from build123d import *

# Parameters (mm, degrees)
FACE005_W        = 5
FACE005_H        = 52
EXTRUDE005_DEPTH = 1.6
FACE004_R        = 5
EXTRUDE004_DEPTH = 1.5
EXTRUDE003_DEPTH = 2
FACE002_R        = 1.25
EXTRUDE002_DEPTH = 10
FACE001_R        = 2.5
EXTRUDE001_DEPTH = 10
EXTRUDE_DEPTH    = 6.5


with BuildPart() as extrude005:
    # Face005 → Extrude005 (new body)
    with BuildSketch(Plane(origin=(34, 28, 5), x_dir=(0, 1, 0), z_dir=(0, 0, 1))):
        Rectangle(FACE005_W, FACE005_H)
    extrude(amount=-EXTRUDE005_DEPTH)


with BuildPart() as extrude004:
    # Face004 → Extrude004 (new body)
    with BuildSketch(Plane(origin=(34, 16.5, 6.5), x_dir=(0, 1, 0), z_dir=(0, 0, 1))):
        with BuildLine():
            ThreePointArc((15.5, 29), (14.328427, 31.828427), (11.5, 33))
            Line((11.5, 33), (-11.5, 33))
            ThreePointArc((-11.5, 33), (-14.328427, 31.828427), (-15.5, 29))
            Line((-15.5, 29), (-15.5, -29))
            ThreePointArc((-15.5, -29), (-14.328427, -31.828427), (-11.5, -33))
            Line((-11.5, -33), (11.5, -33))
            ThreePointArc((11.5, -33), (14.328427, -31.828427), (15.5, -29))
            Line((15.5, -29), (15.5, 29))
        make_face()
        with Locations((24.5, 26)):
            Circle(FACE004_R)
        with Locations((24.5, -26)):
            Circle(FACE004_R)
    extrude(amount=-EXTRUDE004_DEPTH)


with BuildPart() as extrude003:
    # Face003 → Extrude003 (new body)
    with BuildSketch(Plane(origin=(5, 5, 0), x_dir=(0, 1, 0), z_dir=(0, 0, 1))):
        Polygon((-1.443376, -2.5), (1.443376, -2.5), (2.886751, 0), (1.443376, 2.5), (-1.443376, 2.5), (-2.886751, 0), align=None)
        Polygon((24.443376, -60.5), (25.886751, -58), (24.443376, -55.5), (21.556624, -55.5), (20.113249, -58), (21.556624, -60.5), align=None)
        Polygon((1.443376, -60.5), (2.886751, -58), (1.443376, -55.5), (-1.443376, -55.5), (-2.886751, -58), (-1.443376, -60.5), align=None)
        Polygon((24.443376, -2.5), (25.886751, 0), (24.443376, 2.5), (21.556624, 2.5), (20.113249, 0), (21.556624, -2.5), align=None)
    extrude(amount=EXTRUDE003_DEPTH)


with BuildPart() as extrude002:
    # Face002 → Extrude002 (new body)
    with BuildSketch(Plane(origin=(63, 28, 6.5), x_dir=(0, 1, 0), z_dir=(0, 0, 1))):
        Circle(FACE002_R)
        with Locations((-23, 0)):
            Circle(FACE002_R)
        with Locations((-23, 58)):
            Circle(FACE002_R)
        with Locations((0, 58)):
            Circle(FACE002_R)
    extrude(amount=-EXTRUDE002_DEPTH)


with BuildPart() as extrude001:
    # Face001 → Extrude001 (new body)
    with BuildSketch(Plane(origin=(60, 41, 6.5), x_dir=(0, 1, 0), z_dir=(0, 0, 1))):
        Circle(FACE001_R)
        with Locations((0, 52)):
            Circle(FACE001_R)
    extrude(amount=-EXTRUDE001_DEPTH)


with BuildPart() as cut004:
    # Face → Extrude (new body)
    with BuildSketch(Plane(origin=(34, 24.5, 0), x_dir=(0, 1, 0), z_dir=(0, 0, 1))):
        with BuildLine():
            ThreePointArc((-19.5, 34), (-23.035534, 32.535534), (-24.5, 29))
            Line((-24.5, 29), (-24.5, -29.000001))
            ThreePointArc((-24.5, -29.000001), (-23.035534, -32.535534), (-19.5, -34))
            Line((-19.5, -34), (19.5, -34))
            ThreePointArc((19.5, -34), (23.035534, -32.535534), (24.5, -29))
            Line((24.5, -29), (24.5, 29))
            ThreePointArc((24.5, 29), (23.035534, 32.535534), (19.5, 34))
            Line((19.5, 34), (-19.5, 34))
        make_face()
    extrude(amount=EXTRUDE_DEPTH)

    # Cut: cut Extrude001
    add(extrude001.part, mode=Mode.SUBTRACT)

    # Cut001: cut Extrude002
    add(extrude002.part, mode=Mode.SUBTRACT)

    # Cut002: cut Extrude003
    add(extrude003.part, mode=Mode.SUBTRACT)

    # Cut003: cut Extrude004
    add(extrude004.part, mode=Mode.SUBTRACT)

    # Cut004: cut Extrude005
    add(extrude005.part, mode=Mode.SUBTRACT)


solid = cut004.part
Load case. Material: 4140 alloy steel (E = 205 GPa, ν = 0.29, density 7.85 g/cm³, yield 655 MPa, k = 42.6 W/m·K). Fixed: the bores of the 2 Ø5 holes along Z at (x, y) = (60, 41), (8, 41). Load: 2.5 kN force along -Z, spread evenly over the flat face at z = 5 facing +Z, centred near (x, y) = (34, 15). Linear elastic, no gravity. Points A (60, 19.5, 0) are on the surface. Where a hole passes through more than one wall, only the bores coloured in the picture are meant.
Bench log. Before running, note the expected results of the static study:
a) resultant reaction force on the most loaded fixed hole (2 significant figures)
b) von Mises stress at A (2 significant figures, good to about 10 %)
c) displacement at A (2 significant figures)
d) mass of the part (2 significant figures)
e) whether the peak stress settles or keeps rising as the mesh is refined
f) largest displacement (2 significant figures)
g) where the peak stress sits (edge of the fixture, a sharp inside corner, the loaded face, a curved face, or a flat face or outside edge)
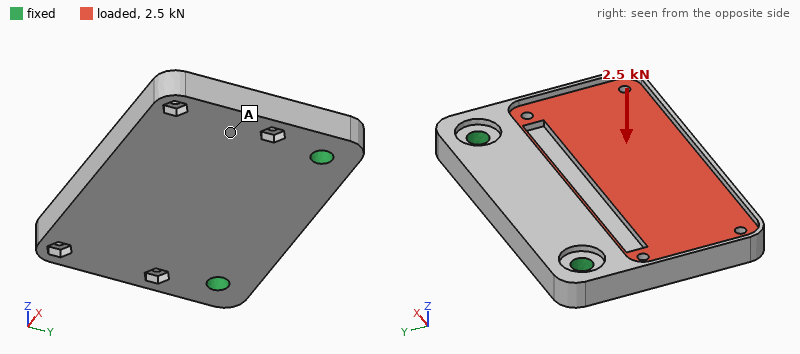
1.3 kN
59 MPa
0.100 mm
140 g
keeps rising
0.29 mm
edge of the fixture
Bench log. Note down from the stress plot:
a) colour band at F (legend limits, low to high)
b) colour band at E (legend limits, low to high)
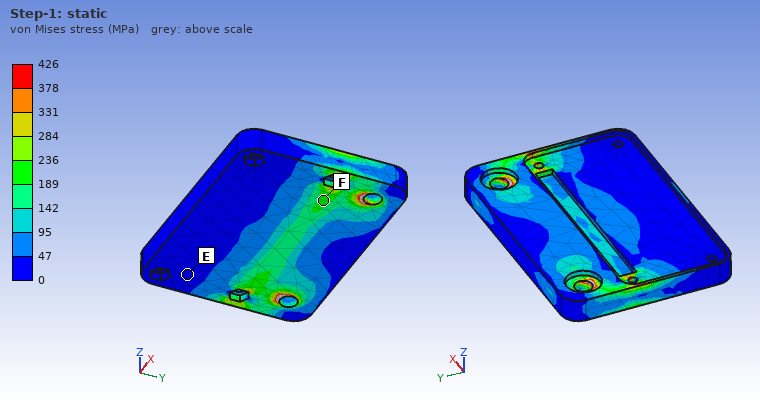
189 to 236 MPa
0 to 47 MPa
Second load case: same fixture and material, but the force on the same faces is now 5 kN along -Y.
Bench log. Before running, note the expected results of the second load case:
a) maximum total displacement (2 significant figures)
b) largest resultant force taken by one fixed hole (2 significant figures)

86 µm
2.5 kN
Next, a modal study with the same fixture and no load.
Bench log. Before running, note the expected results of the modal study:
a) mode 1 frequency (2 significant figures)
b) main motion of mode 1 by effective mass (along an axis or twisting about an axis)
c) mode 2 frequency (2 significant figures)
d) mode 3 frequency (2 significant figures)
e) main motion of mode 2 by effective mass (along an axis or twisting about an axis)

2100 Hz
along Z
4300 Hz
8200 Hz
twisting about Y
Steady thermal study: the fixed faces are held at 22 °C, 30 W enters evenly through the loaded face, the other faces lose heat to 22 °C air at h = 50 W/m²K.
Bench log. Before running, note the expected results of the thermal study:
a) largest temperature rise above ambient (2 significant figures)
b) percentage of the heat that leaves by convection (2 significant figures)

52 K
33 %
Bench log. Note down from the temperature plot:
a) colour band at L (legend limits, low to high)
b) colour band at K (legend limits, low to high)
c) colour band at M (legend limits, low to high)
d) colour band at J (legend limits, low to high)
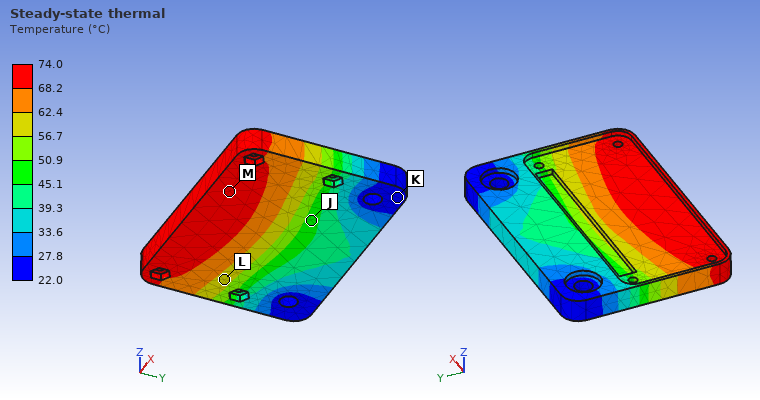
56.7 to 62.4 °C
22.0 to 27.8 °C
68.2 to 74.0 °C
45.1 to 50.9 °C
